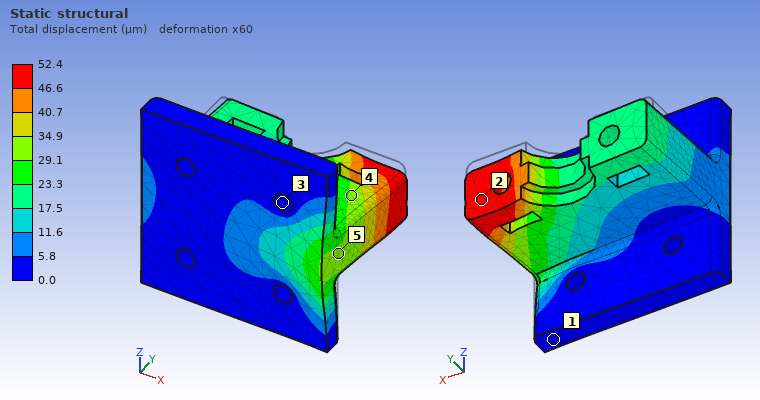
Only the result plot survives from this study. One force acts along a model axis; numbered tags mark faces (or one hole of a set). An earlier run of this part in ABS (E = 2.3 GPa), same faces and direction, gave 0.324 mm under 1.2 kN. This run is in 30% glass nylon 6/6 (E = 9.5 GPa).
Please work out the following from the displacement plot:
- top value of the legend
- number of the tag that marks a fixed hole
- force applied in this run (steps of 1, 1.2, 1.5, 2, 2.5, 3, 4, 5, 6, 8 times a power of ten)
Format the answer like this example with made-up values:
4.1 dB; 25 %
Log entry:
52.4 µm; 3; 800 N
